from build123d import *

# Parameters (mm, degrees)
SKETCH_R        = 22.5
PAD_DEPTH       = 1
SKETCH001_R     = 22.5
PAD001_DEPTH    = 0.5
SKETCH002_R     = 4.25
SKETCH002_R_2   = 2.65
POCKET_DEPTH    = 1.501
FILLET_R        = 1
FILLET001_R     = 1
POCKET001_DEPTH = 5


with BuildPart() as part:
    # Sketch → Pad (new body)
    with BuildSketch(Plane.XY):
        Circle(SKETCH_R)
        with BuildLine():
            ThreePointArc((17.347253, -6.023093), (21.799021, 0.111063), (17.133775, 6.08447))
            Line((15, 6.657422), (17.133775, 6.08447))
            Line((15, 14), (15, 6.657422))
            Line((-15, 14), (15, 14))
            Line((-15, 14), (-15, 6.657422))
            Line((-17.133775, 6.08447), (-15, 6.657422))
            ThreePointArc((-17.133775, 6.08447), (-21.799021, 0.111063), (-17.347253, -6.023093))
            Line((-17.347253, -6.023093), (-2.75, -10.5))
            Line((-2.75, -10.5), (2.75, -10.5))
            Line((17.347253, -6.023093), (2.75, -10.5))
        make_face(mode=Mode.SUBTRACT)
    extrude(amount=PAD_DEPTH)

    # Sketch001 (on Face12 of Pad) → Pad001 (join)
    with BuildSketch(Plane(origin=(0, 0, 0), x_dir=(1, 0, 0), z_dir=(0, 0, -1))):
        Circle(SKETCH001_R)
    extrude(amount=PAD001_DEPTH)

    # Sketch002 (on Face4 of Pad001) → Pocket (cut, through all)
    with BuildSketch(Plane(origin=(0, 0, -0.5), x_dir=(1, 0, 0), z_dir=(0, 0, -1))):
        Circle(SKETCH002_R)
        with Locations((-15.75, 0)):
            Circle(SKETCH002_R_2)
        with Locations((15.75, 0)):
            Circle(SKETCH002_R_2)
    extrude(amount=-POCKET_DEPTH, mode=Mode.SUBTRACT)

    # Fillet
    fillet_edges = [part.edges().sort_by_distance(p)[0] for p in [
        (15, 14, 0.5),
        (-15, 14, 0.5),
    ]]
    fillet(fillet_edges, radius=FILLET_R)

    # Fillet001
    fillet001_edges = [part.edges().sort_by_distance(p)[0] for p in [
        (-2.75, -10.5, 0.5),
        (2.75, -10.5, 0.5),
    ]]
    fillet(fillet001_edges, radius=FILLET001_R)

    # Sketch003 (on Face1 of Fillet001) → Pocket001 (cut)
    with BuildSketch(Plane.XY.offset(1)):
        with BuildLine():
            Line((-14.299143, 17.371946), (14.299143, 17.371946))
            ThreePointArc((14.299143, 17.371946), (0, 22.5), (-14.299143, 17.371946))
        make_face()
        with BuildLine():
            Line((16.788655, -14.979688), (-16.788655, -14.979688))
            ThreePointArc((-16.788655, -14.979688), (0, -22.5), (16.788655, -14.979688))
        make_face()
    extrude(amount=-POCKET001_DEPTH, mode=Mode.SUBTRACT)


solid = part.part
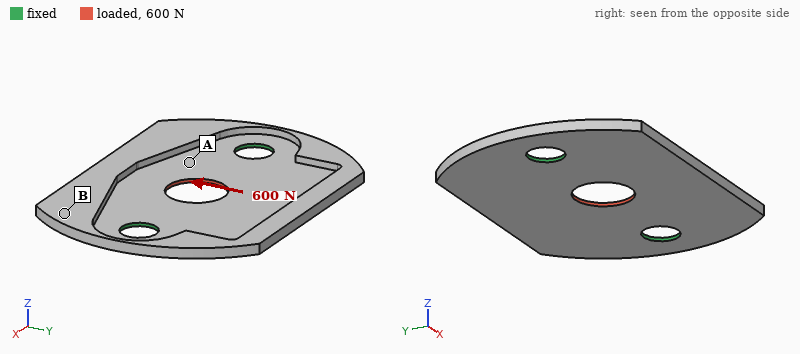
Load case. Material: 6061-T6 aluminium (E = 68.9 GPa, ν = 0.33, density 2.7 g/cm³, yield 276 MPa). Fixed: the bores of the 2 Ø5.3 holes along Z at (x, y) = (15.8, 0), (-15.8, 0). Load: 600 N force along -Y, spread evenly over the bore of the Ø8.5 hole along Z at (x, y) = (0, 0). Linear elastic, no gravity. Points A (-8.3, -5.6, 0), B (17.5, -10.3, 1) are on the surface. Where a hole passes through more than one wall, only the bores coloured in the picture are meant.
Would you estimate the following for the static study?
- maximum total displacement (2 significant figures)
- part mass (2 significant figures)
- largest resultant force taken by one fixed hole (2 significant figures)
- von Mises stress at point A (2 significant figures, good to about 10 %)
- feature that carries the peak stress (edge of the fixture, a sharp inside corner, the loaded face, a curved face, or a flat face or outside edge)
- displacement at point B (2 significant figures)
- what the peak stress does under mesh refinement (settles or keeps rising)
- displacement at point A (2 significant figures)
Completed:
31 µm
3.0 g
300 N
41 MPa
edge of the fixture
5.8 µm
keeps rising
17 µm
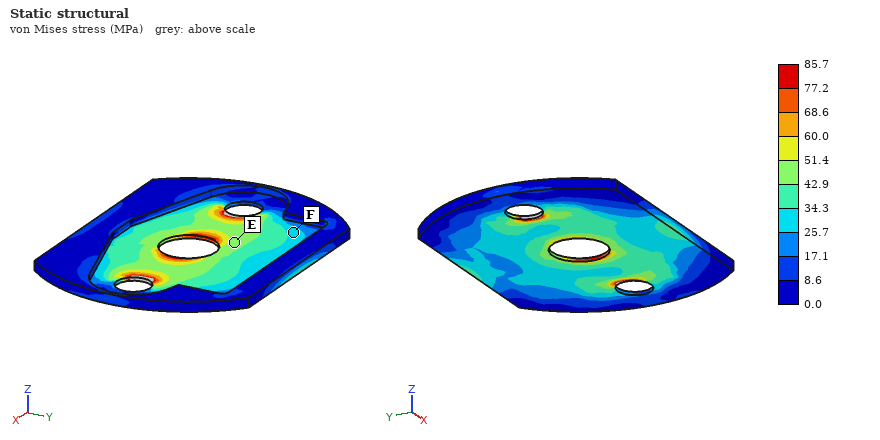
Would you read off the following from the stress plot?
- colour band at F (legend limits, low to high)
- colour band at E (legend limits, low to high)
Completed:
25.7 to 34.3 MPa
42.9 to 51.4 MPa
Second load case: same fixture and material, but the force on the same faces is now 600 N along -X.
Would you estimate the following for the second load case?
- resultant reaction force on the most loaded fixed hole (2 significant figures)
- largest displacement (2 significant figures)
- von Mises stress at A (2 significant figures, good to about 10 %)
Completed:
300 N
9.1 µm
27 MPa
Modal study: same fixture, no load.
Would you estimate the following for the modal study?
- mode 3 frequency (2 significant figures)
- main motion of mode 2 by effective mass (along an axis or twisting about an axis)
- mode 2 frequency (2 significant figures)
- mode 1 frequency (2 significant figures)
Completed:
3600 Hz
along Z
2100 Hz
1700 Hz
